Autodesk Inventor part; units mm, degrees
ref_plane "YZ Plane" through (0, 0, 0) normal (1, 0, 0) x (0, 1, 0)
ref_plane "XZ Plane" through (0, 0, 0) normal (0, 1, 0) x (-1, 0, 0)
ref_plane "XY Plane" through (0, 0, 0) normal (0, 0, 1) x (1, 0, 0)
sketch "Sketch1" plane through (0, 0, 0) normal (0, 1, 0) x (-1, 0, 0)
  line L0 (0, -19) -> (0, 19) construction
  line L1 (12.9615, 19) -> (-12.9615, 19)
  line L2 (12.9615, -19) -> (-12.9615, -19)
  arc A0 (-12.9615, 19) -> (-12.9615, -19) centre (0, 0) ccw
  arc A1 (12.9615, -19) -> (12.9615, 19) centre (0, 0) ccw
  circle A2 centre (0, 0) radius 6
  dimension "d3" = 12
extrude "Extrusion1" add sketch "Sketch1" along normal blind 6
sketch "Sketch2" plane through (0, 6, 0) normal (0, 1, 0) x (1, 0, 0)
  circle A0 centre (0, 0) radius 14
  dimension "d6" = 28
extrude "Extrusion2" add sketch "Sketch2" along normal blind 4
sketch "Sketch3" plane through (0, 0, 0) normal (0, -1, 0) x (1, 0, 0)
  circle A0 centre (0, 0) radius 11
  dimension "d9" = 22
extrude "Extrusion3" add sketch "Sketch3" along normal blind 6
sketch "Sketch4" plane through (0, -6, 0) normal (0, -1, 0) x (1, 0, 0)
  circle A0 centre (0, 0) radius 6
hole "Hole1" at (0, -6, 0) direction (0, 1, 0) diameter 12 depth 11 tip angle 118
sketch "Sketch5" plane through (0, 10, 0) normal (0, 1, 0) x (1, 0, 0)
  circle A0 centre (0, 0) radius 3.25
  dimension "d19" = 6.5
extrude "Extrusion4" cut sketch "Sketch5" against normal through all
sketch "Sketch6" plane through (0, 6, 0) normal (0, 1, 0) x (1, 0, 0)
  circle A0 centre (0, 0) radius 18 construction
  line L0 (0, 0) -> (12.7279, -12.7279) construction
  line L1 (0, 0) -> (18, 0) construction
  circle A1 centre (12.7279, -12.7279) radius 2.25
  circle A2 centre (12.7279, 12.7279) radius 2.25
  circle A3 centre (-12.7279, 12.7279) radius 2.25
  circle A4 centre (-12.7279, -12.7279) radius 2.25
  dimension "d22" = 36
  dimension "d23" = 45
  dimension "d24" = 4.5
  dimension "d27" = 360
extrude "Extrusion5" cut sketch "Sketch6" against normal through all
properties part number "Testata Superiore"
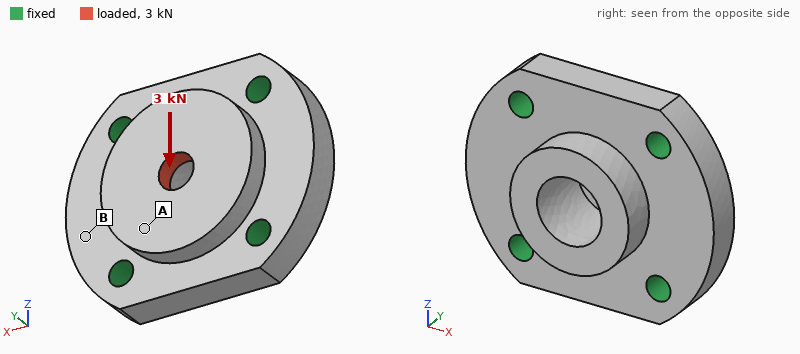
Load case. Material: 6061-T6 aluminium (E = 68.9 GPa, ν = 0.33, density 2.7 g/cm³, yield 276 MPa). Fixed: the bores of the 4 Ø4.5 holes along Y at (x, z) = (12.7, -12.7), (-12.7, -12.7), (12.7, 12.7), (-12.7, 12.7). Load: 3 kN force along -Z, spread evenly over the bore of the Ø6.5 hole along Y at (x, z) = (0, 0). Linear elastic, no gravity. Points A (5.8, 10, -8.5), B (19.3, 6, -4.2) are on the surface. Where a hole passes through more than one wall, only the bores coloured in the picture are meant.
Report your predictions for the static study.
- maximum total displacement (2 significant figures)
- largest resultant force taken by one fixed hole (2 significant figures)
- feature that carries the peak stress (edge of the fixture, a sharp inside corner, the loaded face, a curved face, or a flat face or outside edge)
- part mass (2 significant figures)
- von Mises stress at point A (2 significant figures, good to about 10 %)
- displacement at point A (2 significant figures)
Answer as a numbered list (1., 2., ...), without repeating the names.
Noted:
1. 7.3 µm
2. 870 N
3. the loaded face
4. 32 g
5. 14 MPa
6. 3.4 µm
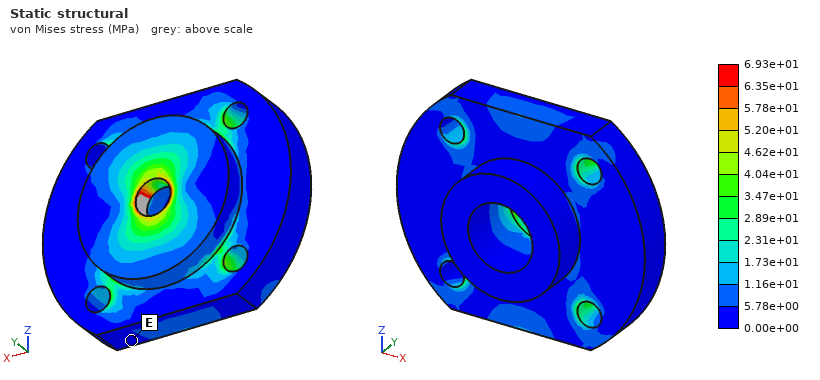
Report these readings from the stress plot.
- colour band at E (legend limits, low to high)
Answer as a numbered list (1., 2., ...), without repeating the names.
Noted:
1. 0.00e+00 to 5.78e+00 MPa
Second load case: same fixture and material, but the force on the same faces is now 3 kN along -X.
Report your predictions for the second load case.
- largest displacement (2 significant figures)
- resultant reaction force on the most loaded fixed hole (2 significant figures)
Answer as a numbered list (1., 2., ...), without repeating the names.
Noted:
1. 7.1 µm
2. 850 N
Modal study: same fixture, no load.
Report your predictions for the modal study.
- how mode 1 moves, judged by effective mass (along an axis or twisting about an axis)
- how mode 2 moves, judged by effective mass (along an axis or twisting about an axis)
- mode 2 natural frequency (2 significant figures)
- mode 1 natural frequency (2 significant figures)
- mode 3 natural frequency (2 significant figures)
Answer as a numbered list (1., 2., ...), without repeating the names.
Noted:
1. along Y
2. twisting about Z
3. 33 kHz
4. 31 kHz
5. 37 kHz
